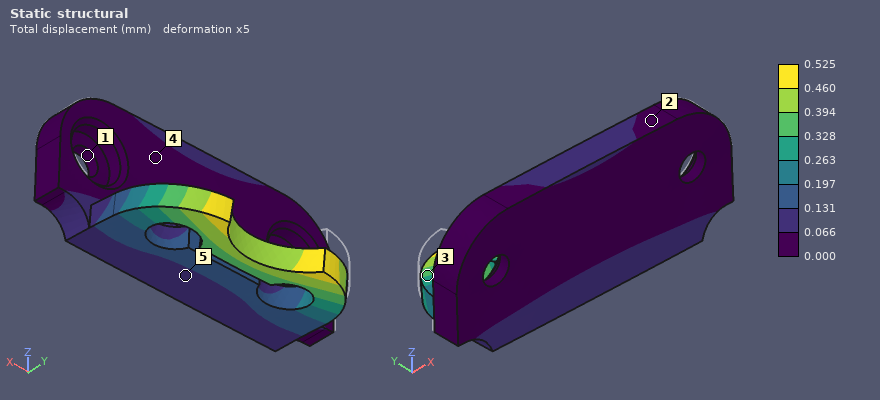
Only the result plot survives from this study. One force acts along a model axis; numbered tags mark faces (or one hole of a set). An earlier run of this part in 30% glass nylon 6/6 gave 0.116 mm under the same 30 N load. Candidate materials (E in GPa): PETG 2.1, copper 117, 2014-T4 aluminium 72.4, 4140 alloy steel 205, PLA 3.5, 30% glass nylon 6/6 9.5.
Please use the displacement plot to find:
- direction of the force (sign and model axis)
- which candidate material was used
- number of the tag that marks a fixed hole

-Z
PETG
1
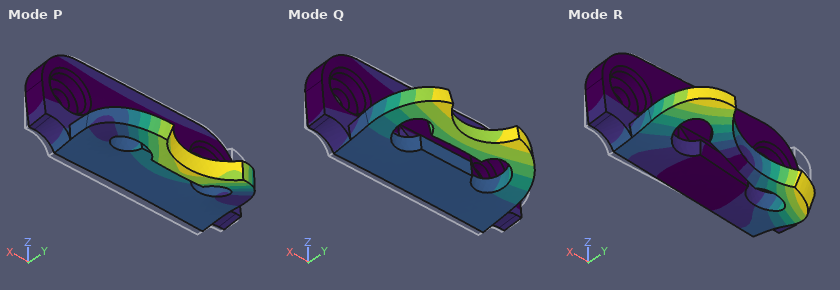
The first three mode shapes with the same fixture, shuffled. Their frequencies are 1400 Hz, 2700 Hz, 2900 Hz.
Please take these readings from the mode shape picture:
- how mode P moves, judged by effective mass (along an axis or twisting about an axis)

along Y
